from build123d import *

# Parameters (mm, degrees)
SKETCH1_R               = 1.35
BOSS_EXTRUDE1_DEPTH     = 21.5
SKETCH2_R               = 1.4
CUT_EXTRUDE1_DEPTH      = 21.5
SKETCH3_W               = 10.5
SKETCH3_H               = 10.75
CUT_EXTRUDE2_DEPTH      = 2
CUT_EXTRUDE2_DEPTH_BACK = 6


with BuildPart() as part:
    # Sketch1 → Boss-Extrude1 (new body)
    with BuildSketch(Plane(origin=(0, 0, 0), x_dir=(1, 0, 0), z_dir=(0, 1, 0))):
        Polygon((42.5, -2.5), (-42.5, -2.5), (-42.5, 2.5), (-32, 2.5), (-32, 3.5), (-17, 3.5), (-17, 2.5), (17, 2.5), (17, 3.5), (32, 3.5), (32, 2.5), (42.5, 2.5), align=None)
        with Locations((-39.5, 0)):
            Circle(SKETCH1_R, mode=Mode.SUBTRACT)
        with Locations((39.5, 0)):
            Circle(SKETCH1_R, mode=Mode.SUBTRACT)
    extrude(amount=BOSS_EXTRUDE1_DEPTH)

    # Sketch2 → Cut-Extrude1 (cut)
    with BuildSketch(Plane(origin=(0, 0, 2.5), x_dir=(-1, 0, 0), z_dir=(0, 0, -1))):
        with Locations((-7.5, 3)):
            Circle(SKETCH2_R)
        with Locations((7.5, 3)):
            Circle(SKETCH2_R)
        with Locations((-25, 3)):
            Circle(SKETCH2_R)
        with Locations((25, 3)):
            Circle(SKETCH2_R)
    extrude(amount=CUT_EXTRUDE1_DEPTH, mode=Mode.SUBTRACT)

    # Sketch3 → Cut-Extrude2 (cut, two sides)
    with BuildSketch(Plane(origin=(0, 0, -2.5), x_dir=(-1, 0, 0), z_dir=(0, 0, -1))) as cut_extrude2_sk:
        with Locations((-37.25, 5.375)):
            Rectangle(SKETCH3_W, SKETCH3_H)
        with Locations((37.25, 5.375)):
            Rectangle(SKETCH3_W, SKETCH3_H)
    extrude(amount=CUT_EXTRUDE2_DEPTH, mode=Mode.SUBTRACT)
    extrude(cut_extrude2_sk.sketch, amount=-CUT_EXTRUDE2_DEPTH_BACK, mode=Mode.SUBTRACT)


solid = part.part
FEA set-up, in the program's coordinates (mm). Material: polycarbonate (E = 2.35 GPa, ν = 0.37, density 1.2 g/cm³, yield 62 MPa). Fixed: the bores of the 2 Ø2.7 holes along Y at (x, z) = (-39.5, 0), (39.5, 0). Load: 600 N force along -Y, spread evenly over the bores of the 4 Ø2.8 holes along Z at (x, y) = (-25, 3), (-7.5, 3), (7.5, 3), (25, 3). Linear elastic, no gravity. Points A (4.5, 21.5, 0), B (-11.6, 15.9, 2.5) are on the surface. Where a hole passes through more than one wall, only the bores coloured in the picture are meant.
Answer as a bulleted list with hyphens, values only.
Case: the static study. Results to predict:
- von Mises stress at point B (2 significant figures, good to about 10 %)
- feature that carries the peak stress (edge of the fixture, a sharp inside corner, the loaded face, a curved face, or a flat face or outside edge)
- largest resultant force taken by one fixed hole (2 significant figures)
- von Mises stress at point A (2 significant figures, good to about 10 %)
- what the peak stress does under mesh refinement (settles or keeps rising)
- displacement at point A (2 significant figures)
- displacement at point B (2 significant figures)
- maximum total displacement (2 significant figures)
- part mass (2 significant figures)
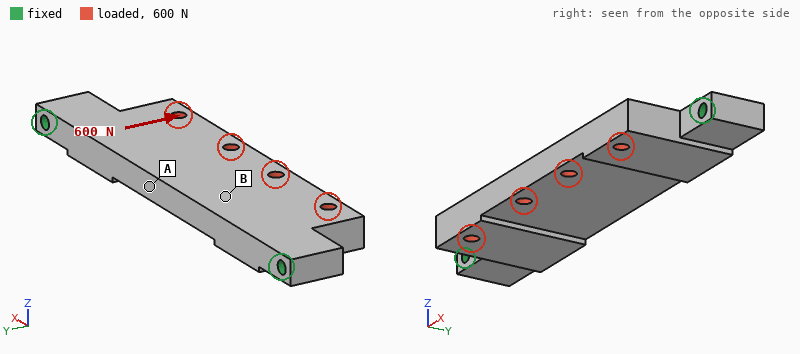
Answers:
- 2.7 MPa
- edge of the fixture
- 360 N
- 7.4 MPa
- keeps rising
- 0.28 mm
- 0.26 mm
- 0.29 mm
- 10 g
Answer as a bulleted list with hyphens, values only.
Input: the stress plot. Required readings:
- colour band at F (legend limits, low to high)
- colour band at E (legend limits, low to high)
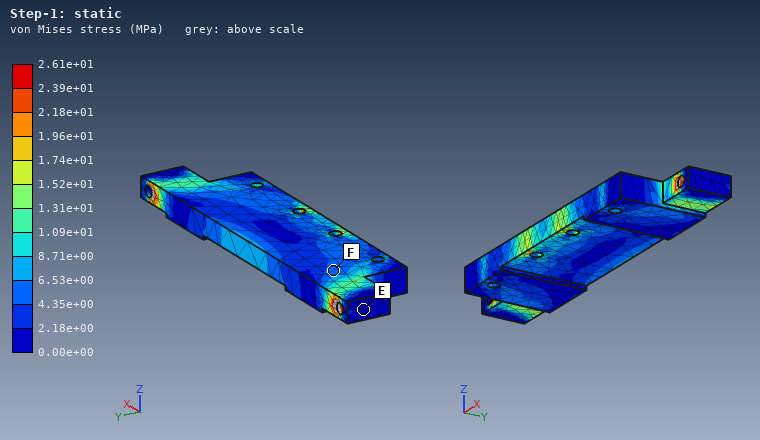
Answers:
- 4.35e+00 to 6.53e+00 MPa
- 0.00e+00 to 2.18e+00 MPa
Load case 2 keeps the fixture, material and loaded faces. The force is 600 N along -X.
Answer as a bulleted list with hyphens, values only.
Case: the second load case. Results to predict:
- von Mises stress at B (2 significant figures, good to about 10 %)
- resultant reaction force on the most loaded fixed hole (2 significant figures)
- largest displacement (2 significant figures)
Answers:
- 2.1 MPa
- 320 N
- 83 µm
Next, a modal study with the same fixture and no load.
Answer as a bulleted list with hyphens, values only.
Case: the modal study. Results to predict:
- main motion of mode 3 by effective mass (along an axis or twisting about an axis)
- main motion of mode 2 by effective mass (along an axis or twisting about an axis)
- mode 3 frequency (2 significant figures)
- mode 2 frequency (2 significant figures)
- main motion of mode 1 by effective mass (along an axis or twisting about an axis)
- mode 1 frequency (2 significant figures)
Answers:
- twisting about Y
- twisting about X
- 2400 Hz
- 1900 Hz
- along Z
- 880 Hz
